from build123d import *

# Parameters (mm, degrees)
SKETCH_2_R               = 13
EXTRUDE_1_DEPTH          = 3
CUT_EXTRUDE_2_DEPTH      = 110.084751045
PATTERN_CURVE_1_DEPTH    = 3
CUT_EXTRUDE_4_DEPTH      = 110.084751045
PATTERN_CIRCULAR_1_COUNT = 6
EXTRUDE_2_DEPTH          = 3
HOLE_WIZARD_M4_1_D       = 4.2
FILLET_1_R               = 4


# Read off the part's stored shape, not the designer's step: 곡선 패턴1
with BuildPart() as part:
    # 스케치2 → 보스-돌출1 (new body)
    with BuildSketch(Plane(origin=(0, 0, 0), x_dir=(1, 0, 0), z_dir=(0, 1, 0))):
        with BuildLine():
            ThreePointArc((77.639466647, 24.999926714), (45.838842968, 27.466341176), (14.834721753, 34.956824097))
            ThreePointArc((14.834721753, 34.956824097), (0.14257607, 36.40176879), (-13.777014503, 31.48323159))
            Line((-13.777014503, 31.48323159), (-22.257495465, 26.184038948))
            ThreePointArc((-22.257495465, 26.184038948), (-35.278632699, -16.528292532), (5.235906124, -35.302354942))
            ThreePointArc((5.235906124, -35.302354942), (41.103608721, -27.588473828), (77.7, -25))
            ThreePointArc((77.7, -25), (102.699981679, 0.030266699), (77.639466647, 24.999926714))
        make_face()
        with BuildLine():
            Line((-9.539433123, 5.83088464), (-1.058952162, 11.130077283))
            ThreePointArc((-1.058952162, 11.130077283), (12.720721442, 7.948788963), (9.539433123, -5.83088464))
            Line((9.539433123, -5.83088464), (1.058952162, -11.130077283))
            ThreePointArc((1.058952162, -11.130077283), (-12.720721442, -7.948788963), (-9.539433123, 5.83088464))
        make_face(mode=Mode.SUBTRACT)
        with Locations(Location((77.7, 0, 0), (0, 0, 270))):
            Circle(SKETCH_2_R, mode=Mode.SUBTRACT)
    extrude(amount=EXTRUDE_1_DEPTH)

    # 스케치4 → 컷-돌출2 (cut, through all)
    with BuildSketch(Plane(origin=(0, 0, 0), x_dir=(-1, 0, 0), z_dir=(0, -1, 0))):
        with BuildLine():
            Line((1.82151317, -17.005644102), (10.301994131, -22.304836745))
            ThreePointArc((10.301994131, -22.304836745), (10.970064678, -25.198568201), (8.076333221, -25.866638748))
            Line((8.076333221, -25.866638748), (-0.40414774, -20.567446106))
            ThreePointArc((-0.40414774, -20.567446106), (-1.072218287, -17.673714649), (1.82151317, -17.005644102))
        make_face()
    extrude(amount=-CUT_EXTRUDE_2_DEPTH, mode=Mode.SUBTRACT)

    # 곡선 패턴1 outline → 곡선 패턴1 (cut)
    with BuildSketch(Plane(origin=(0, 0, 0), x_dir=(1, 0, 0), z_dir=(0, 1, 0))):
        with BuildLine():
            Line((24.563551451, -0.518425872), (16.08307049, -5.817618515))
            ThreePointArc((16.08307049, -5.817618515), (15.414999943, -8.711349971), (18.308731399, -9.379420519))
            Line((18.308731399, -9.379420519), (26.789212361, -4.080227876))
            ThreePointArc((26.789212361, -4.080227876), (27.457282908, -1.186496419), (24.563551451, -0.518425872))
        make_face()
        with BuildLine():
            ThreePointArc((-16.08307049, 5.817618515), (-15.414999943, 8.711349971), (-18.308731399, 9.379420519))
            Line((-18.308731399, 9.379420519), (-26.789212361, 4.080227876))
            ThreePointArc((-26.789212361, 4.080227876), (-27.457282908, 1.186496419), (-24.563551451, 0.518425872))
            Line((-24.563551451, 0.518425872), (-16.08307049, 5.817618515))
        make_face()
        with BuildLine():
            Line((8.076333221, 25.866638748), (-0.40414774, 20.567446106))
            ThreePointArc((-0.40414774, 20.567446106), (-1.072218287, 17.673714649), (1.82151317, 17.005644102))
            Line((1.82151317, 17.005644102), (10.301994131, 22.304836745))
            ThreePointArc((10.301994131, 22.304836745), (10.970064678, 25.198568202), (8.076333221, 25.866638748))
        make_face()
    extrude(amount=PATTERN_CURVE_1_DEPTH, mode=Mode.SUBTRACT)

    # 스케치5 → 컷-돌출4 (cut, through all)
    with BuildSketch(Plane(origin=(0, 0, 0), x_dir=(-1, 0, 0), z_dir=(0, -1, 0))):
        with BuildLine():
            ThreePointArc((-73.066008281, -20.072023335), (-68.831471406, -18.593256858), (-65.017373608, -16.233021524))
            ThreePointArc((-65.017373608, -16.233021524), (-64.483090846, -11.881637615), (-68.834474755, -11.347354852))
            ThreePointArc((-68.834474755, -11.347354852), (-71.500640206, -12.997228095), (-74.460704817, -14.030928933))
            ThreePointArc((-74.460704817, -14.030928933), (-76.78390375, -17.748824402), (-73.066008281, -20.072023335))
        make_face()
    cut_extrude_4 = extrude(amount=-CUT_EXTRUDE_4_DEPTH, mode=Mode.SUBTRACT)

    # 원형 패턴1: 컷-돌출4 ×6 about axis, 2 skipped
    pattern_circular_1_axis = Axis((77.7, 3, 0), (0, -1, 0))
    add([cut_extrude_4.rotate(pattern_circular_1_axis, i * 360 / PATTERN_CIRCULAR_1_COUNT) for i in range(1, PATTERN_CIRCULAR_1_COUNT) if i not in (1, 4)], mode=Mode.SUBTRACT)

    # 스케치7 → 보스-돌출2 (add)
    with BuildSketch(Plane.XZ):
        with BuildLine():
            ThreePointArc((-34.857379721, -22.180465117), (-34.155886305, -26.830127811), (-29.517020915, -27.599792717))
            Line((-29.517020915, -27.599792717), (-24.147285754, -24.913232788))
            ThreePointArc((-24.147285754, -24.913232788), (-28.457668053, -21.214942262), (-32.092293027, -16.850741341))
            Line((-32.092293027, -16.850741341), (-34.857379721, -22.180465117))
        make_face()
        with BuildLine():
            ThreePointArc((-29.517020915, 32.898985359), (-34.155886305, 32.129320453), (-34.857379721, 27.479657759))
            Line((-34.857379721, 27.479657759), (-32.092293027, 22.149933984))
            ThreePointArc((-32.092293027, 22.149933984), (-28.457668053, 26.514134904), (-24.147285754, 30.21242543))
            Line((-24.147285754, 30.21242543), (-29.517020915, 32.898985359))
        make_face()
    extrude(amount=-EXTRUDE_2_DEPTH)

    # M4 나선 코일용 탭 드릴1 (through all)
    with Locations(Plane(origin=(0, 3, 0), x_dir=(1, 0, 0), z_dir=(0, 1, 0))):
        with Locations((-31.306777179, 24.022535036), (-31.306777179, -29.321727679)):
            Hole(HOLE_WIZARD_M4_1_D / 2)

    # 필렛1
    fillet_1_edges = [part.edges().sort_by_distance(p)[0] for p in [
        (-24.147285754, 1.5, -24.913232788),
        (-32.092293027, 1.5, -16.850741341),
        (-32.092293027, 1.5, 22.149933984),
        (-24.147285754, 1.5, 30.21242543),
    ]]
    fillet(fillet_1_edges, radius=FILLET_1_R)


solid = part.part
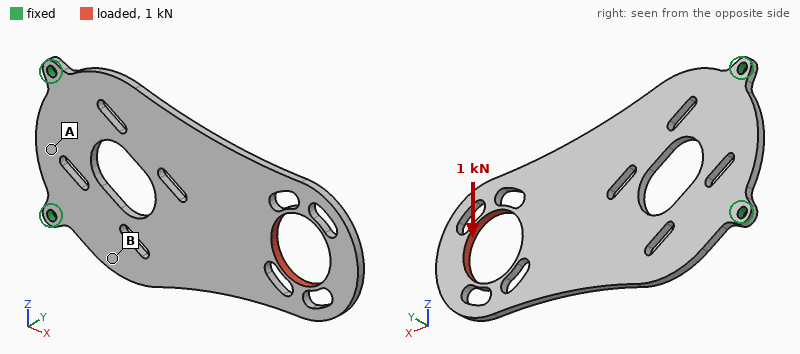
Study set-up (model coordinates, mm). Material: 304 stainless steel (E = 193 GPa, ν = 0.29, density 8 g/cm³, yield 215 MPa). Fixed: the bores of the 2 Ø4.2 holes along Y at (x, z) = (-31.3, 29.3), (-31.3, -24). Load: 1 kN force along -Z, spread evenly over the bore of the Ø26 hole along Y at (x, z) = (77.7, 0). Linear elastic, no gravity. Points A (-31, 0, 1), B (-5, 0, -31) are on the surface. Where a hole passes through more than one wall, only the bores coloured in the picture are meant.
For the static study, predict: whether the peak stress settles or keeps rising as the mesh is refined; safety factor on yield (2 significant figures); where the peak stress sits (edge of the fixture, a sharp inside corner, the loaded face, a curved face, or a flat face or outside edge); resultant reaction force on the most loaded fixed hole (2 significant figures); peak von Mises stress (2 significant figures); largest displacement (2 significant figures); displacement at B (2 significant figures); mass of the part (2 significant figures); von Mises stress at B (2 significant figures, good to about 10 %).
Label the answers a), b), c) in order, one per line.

a) settles
b) 0.97
c) a curved face
d) 2.2 kN
e) 220 MPa
f) 0.10 mm
g) 0.018 mm
h) 150 g
i) 35 MPa
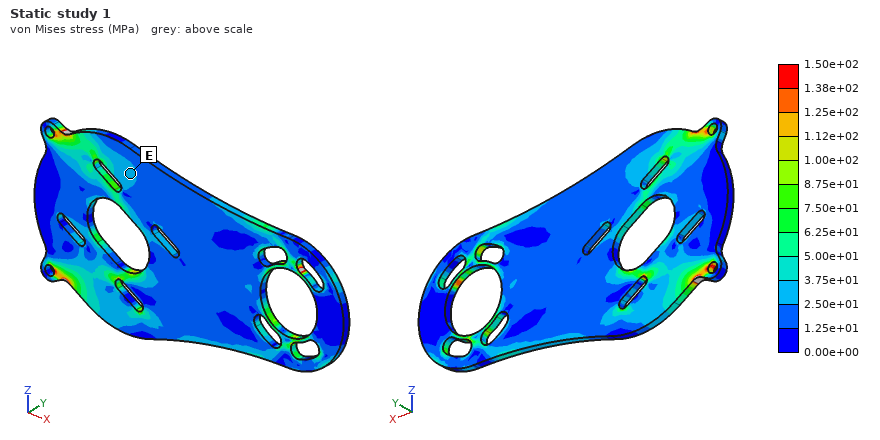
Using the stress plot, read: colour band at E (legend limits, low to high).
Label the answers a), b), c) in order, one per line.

a) 2.50e+01 to 3.75e+01 MPa
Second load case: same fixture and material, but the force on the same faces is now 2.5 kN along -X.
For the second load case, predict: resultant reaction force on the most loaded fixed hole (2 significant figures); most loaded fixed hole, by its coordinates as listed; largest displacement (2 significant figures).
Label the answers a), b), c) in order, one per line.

a) 1.4 kN
b) (-31.3, -24)
c) 33 µm
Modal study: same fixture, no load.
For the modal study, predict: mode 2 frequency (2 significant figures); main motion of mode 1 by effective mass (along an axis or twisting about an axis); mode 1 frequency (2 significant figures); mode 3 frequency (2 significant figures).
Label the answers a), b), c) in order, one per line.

a) 760 Hz
b) along Y
c) 150 Hz
d) 810 Hz
